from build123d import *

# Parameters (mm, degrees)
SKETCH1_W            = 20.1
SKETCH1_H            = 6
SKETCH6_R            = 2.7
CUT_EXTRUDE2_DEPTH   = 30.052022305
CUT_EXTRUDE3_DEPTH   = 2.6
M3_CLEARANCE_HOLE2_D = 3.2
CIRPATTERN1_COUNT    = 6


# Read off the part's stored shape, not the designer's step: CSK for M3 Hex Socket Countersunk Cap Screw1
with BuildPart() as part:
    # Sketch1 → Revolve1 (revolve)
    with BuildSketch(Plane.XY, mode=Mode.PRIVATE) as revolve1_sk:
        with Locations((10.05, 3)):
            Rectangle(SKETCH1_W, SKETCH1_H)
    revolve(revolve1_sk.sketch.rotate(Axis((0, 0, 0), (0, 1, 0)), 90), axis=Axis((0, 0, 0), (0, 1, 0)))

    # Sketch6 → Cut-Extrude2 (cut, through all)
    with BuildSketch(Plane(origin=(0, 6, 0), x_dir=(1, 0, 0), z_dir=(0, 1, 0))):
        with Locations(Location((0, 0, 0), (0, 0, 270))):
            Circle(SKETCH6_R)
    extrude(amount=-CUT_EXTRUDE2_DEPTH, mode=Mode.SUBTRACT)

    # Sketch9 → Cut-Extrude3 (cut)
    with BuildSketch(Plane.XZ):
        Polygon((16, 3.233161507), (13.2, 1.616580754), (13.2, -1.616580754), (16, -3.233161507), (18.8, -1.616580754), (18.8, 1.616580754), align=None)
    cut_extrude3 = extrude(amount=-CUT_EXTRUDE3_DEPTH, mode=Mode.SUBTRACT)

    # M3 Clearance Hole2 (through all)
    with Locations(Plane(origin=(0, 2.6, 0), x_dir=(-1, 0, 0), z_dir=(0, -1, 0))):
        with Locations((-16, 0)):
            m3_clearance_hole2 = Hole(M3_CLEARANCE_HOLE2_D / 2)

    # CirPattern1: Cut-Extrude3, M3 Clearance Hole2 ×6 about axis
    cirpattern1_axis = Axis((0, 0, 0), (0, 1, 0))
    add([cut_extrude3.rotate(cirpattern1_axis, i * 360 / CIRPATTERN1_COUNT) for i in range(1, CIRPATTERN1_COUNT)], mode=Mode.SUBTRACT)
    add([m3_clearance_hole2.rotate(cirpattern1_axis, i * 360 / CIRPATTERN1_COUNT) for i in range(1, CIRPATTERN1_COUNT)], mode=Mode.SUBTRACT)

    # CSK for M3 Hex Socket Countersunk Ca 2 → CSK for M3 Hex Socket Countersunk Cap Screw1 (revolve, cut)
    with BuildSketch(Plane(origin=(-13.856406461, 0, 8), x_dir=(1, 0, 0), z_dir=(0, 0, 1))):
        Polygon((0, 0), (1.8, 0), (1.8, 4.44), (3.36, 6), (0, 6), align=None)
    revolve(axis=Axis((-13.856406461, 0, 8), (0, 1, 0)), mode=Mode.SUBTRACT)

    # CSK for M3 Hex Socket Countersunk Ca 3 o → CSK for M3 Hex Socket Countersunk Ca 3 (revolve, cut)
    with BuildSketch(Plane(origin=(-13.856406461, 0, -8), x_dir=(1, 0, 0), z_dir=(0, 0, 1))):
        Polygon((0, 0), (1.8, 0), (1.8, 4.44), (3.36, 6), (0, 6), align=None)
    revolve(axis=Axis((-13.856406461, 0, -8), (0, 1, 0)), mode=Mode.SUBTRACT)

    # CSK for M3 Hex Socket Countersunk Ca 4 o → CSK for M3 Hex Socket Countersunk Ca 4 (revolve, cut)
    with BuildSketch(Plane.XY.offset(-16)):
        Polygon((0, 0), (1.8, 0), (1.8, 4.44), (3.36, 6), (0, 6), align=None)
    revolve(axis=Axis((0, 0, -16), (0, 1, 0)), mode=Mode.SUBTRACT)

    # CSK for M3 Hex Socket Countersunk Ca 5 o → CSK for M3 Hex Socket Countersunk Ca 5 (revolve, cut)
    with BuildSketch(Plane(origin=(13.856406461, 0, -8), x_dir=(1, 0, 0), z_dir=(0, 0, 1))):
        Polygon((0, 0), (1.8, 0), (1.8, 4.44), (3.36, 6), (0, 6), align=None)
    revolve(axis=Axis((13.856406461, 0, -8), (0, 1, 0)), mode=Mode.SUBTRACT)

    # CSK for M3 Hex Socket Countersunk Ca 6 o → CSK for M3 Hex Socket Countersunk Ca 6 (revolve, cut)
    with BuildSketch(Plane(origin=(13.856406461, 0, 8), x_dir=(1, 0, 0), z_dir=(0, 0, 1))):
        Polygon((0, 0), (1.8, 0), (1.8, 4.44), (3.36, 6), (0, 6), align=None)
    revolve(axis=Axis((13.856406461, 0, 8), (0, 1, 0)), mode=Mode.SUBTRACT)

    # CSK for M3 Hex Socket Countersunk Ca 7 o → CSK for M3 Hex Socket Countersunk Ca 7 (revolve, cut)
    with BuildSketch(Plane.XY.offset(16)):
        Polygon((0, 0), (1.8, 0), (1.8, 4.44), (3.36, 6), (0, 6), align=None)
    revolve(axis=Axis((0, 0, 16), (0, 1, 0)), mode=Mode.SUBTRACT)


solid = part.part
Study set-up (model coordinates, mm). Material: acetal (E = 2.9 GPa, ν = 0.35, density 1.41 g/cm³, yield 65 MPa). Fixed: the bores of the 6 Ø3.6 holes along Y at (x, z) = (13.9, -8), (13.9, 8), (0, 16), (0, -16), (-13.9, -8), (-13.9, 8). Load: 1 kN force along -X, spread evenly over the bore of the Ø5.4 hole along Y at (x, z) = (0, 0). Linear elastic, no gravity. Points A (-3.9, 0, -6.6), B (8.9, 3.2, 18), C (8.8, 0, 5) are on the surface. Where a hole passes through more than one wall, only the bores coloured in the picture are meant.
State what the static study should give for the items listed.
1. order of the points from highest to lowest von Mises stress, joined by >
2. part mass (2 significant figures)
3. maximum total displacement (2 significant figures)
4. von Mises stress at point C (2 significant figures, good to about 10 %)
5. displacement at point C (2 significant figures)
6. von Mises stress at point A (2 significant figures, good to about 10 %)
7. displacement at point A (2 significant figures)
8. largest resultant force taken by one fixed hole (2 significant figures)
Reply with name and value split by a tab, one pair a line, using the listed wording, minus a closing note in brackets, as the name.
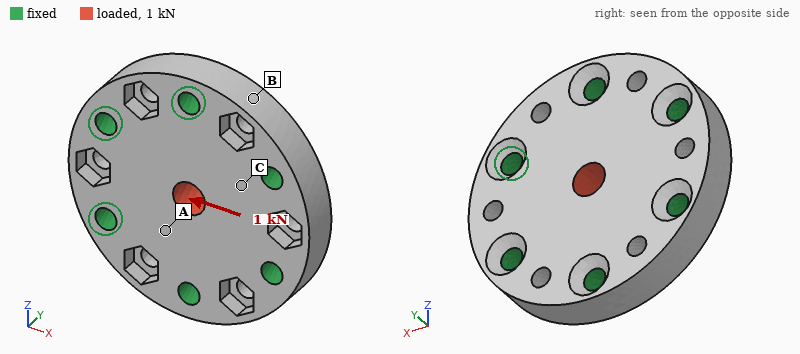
order of the points from highest to lowest von Mises stress, joined by >	C > A > B
part mass	9.0 g
maximum total displacement	31 µm
von Mises stress at point C	6.4 MPa
displacement at point C	9.6 µm
von Mises stress at point A	3.7 MPa
displacement at point A	13 µm
largest resultant force taken by one fixed hole	240 N
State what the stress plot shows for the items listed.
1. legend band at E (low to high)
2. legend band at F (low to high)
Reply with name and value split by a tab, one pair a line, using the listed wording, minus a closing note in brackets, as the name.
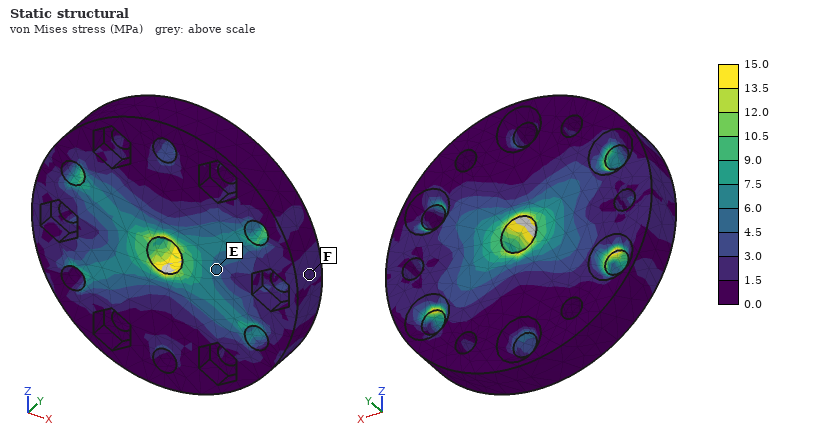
legend band at E	4.5 to 6.0 MPa
legend band at F	1.5 to 3.0 MPa
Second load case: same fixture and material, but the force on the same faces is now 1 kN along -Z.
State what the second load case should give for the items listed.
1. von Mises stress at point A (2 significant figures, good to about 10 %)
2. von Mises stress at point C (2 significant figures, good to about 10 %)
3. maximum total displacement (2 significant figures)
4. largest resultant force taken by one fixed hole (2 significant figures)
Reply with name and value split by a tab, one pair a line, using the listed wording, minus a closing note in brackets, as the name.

von Mises stress at point A	4.8 MPa
von Mises stress at point C	3.8 MPa
maximum total displacement	31 µm
largest resultant force taken by one fixed hole	280 N
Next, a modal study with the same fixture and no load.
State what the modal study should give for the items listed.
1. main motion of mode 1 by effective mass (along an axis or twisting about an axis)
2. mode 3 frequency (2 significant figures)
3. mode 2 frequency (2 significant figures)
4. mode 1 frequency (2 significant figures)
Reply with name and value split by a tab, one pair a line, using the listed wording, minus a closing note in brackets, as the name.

main motion of mode 1 by effective mass	along Y
mode 3 frequency	18 kHz
mode 2 frequency	18 kHz
mode 1 frequency	11 kHz
